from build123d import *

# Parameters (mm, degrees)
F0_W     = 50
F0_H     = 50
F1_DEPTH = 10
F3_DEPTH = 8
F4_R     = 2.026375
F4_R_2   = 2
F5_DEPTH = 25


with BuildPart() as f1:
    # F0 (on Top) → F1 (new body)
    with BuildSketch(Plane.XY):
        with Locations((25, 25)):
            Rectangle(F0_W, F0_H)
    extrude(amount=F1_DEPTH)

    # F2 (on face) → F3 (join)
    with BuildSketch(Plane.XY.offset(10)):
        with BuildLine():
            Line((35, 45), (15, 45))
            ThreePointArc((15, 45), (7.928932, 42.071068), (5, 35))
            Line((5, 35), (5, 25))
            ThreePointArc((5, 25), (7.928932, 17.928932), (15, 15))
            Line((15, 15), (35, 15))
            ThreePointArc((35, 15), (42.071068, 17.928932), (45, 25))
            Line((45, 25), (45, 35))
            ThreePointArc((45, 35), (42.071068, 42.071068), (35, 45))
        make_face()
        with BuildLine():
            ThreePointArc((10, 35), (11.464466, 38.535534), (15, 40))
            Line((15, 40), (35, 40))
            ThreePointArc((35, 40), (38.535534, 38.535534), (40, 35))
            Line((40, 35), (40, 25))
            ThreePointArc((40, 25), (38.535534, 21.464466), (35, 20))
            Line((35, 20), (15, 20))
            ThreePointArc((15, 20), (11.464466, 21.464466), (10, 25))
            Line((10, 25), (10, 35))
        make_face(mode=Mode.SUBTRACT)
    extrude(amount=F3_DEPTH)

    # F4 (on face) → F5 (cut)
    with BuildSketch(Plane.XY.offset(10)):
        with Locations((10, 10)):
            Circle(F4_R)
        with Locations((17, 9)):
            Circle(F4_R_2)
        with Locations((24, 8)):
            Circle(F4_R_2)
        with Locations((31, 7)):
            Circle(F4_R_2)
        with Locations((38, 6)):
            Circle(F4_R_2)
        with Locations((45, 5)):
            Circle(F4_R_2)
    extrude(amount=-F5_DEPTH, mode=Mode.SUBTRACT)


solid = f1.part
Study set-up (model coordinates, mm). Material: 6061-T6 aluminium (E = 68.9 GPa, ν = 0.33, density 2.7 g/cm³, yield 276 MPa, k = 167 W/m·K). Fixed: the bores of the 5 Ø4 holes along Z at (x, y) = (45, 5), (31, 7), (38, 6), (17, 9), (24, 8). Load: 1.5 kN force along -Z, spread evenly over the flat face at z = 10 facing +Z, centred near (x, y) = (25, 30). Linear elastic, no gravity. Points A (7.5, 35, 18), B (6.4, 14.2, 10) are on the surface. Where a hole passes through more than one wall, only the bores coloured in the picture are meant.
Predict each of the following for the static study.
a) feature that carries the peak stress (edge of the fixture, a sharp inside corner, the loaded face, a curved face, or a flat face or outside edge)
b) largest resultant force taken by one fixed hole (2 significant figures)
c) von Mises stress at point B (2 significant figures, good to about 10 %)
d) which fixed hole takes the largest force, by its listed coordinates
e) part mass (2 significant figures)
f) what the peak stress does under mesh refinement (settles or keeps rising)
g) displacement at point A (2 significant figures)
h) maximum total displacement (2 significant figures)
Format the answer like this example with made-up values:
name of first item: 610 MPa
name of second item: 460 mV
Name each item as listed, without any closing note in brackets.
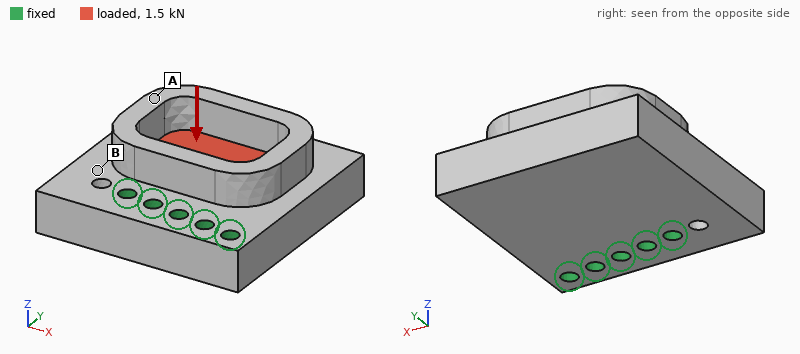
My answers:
feature that carries the peak stress: edge of the fixture
largest resultant force taken by one fixed hole: 640 N
von Mises stress at point B: 15 MPa
which fixed hole takes the largest force, by its listed coordinates: (17, 9)
part mass: 77 g
what the peak stress does under mesh refinement: keeps rising
displacement at point A: 33 µm
maximum total displacement: 48 µm
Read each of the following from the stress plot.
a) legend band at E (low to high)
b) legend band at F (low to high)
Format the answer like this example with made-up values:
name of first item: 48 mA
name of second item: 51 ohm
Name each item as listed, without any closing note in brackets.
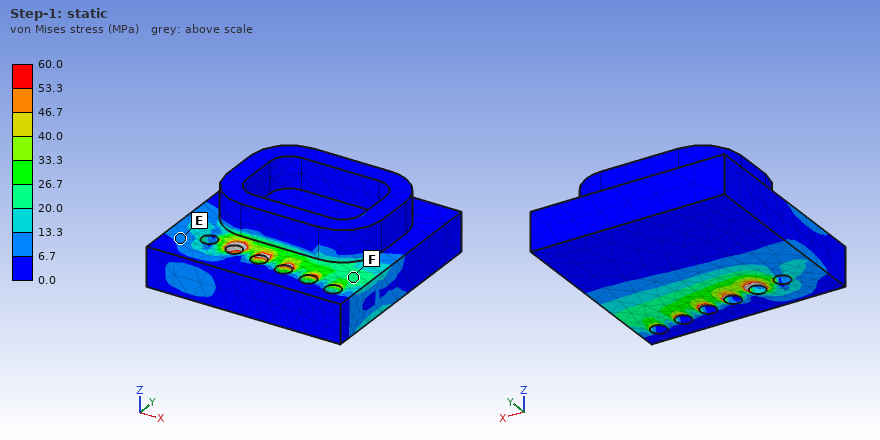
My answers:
legend band at E: 6.7 to 13.3 MPa
legend band at F: 20.0 to 26.7 MPa
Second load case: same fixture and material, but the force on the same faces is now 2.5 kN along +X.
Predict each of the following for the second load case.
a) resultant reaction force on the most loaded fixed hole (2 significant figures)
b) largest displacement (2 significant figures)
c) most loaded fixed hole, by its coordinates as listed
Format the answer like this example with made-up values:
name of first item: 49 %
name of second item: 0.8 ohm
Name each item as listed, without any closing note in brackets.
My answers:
resultant reaction force on the most loaded fixed hole: 2.1 kN
largest displacement: 19 µm
most loaded fixed hole, by its coordinates as listed: (17, 9)
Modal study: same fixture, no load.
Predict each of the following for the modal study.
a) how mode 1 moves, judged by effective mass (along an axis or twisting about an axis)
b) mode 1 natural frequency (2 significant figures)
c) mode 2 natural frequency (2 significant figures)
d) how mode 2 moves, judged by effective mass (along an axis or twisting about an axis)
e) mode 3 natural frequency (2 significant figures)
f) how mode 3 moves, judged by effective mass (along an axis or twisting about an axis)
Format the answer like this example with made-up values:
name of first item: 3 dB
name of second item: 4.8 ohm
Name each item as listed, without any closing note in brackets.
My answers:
how mode 1 moves, judged by effective mass: along Z
mode 1 natural frequency: 4100 Hz
mode 2 natural frequency: 7700 Hz
how mode 2 moves, judged by effective mass: twisting about Y
mode 3 natural frequency: 9500 Hz
how mode 3 moves, judged by effective mass: along X
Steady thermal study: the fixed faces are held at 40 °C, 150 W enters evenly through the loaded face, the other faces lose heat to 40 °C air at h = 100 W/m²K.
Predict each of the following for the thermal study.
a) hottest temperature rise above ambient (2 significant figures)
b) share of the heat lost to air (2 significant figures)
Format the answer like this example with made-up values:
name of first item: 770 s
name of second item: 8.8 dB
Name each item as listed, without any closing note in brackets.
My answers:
hottest temperature rise above ambient: 42 K
share of the heat lost to air: 12 %
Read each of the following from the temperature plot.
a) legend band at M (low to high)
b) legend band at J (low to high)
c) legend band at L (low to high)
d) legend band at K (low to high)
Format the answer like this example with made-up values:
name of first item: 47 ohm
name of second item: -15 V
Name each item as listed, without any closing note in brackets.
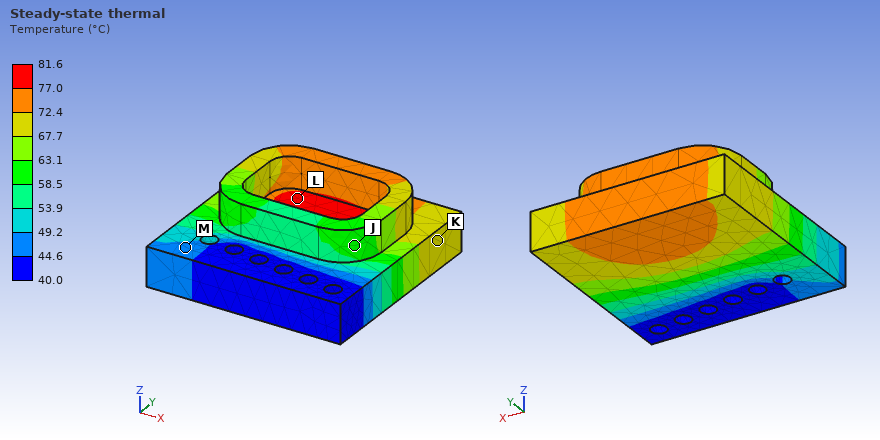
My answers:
legend band at M: 44.6 to 49.2 °C
legend band at J: 58.5 to 63.1 °C
legend band at L: 77.0 to 81.6 °C
legend band at K: 67.7 to 72.4 °C
